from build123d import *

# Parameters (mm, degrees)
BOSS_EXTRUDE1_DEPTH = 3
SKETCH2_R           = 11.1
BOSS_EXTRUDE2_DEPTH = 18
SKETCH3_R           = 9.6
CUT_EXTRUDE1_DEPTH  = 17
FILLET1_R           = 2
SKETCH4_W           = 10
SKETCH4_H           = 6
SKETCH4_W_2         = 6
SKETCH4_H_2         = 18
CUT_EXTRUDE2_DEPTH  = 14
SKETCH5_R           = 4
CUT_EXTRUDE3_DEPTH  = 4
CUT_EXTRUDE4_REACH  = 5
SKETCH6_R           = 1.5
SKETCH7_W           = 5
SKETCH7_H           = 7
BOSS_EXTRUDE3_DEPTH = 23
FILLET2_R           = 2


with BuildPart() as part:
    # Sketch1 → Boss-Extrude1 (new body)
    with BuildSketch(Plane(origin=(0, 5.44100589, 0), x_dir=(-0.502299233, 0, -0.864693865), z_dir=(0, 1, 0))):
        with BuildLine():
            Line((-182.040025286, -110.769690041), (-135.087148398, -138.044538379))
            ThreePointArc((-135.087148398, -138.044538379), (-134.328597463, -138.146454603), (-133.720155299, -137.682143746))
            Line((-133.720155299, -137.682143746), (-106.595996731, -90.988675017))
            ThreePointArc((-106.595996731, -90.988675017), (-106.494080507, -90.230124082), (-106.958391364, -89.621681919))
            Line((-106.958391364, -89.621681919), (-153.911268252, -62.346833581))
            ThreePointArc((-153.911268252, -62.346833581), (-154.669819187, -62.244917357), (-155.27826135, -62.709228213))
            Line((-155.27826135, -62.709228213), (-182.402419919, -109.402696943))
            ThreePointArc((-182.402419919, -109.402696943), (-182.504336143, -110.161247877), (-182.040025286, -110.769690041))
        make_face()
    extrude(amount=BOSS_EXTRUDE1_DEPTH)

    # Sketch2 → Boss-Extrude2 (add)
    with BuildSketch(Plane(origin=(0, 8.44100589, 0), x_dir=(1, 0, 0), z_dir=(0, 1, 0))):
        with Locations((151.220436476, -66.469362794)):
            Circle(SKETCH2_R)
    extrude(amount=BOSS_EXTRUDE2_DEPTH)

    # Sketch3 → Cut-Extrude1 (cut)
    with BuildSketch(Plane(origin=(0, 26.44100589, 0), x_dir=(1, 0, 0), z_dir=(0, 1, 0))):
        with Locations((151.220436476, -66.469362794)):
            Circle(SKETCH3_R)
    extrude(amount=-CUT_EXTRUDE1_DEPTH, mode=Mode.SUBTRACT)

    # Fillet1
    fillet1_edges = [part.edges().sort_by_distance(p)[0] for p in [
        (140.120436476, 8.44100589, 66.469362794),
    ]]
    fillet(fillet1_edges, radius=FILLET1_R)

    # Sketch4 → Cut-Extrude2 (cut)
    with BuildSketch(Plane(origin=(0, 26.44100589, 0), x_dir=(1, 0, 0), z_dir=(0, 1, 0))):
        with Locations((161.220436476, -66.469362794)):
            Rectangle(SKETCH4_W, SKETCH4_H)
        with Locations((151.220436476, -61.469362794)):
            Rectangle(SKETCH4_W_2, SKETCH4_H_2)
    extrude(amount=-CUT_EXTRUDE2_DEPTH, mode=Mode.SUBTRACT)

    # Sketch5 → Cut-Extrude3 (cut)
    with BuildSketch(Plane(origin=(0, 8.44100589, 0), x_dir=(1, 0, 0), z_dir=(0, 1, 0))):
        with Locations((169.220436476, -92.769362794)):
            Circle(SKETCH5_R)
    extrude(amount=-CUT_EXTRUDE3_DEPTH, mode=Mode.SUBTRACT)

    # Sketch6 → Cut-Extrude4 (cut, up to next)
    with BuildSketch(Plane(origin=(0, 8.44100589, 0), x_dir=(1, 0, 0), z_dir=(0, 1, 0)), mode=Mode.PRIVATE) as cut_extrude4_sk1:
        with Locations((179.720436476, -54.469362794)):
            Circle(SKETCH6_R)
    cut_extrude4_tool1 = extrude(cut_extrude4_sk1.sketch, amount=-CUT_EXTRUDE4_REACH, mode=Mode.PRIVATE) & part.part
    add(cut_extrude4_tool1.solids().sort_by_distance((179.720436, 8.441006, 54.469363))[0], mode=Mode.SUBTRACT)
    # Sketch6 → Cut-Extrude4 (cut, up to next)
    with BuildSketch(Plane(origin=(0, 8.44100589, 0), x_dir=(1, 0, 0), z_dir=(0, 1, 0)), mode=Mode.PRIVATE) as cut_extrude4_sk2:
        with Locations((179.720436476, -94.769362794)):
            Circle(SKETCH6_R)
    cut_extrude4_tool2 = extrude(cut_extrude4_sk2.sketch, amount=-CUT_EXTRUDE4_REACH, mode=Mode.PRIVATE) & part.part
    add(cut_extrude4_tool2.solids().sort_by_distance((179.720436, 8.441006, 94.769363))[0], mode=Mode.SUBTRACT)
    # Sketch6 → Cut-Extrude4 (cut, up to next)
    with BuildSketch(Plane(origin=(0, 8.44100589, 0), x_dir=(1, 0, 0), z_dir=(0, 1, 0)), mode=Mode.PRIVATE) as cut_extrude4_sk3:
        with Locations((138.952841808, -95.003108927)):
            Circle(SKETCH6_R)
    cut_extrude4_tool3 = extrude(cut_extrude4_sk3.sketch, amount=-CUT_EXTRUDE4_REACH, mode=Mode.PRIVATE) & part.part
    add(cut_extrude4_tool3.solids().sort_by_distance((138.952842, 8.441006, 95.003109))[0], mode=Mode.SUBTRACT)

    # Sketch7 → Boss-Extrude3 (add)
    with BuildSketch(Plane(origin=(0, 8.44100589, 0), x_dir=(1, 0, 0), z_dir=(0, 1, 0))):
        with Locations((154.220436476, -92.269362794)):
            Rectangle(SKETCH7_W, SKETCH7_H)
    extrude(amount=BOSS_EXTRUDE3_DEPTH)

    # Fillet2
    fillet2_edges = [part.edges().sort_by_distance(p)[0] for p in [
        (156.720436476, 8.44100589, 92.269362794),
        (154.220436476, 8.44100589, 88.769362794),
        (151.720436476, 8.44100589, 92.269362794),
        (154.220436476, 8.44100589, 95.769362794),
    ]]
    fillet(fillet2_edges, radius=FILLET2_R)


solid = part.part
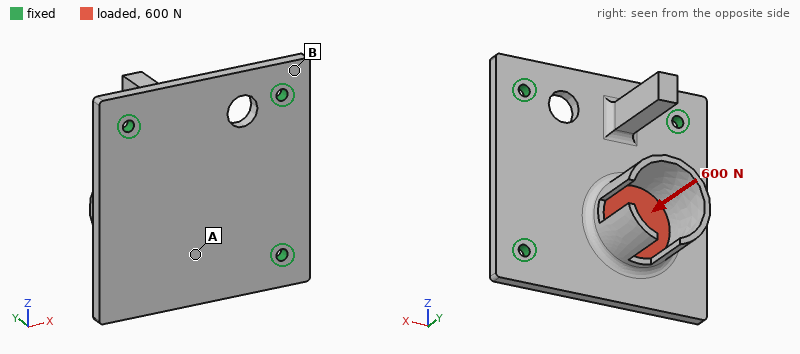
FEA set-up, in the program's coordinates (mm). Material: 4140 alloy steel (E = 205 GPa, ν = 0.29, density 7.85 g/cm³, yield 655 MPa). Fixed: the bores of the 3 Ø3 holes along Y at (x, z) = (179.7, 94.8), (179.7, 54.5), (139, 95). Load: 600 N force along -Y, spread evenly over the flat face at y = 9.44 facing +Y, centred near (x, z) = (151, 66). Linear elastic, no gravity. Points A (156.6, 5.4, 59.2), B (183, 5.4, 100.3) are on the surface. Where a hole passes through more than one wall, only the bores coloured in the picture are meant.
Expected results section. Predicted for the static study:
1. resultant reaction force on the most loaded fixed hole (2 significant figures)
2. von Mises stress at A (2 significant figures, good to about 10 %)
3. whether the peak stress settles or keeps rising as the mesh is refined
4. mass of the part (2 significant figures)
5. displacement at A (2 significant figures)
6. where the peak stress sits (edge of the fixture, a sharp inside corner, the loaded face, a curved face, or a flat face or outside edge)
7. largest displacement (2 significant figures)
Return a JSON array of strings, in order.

["350 N", "45 MPa", "keeps rising", "94 g", "0.058 mm", "edge of the fixture", "0.14 mm"]
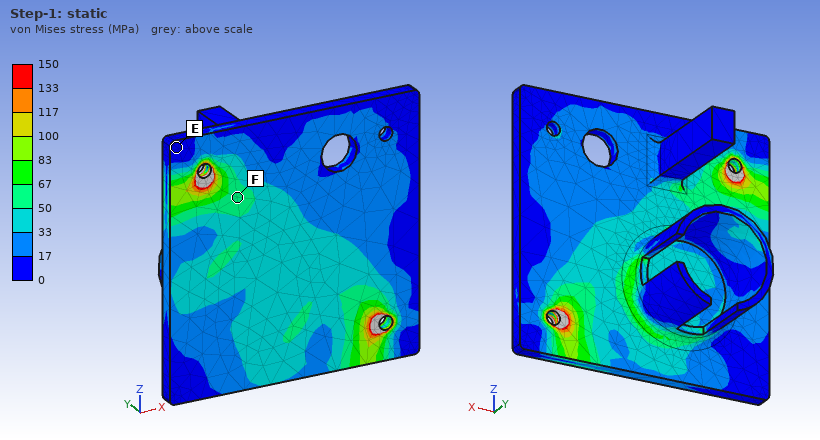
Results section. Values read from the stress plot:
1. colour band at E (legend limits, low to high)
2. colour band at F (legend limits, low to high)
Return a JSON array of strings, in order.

["0 to 17 MPa", "50 to 67 MPa"]
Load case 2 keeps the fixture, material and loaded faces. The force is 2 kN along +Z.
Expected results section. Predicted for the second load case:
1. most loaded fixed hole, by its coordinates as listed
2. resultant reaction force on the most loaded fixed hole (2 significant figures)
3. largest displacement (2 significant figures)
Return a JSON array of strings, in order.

["(139, 95)", "1.1 kN", "60 µm"]
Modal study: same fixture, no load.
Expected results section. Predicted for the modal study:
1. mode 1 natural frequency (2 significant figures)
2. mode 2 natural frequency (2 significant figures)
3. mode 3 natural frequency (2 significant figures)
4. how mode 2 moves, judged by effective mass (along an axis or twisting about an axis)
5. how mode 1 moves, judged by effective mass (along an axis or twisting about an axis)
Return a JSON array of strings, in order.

["1900 Hz", "4900 Hz", "5400 Hz", "along Y", "along Y"]
